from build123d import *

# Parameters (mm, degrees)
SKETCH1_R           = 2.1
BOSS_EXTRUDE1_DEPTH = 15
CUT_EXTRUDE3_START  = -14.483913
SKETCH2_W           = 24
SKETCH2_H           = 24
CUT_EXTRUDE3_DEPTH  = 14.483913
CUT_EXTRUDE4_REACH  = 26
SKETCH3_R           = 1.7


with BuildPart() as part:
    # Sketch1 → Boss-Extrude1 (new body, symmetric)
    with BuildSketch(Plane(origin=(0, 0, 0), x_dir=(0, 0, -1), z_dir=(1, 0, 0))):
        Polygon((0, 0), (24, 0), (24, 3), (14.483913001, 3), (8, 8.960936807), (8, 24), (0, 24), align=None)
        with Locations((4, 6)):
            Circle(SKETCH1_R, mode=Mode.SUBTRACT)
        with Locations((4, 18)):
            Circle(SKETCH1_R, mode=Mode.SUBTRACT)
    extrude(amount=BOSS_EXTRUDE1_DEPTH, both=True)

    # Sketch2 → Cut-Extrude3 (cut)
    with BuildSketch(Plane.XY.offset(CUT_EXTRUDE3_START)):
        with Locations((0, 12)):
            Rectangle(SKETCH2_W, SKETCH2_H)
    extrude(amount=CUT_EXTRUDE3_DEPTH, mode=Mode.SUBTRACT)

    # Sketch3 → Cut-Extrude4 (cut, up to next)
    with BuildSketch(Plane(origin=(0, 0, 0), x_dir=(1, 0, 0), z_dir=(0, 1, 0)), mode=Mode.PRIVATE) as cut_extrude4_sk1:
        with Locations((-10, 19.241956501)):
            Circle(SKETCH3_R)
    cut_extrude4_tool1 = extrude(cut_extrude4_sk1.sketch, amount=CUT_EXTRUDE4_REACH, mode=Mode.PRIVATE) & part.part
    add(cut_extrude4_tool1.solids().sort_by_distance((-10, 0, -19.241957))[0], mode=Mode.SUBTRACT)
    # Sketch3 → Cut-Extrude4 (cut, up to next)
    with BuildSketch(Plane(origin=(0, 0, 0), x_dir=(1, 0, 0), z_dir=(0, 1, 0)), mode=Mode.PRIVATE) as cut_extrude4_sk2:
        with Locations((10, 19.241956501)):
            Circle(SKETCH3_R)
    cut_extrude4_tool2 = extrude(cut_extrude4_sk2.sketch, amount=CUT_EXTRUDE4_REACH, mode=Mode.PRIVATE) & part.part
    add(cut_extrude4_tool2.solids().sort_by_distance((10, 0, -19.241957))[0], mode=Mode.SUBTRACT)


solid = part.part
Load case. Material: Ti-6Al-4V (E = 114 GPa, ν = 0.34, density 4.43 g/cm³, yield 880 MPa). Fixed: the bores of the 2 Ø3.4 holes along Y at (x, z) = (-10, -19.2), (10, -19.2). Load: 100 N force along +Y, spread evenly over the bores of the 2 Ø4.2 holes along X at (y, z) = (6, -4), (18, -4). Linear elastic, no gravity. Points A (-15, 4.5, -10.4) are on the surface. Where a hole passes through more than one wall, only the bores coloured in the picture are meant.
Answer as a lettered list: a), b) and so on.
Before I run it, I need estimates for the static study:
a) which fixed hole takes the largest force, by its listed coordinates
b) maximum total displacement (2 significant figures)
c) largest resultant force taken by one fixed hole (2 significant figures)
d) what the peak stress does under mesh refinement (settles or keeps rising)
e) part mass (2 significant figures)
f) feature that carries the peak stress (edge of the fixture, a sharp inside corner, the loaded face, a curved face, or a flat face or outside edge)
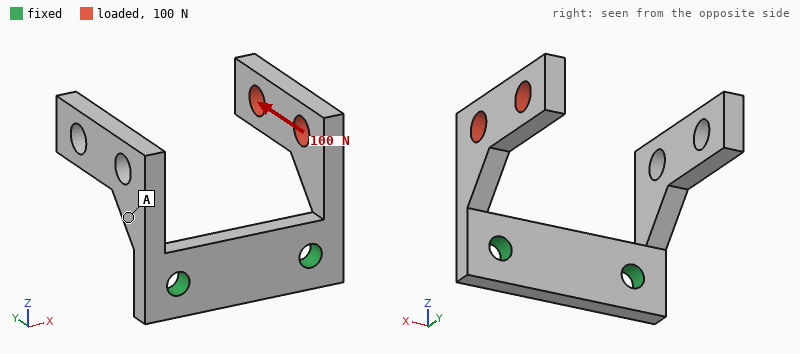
a) (10, -19.2)
b) 0.20 mm
c) 110 N
d) keeps rising
e) 9.0 g
f) a sharp inside corner
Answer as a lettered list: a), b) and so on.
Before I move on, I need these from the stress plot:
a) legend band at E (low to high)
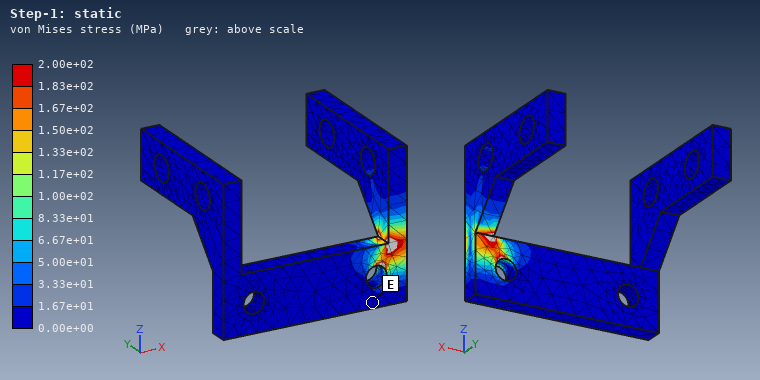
a) 0.00e+00 to 1.67e+01 MPa
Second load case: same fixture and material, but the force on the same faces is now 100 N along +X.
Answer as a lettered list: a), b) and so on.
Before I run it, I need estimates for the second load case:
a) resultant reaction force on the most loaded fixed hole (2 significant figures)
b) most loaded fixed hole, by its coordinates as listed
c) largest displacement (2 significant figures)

a) 84 N
b) (10, -19.2)
c) 0.36 mm
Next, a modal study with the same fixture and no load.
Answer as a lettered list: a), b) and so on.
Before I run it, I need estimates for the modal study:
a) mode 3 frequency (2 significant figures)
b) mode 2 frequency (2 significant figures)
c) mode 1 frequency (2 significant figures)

a) 2400 Hz
b) 2300 Hz
c) 2300 Hz
